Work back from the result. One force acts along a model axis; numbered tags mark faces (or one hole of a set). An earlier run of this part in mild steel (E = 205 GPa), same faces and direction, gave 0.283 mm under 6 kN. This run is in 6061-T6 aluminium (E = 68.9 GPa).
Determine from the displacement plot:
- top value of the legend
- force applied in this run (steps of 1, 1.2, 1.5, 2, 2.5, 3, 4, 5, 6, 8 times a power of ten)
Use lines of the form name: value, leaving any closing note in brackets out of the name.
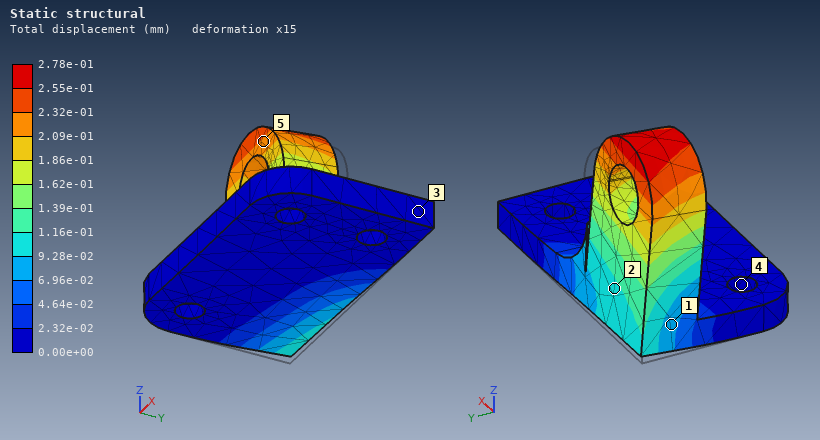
top value of the legend: 2.78e-01 mm
force applied in this run: 2 kN
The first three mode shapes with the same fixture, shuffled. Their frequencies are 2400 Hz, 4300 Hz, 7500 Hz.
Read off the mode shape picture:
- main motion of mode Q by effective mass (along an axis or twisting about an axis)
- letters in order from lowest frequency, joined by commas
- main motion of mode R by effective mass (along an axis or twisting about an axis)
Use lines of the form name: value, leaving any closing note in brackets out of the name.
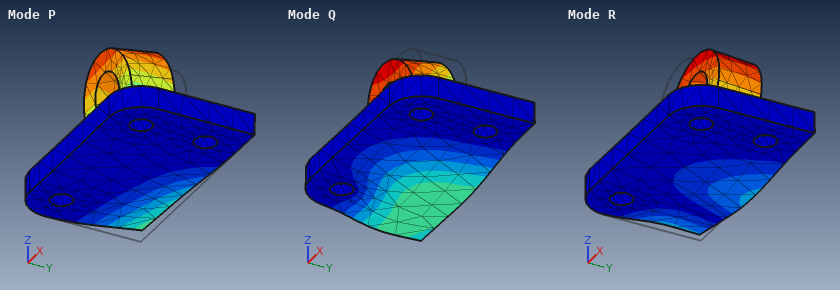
main motion of mode Q by effective mass: along Z
letters in order from lowest frequency, joined by commas: P, R, Q
main motion of mode R by effective mass: along X
